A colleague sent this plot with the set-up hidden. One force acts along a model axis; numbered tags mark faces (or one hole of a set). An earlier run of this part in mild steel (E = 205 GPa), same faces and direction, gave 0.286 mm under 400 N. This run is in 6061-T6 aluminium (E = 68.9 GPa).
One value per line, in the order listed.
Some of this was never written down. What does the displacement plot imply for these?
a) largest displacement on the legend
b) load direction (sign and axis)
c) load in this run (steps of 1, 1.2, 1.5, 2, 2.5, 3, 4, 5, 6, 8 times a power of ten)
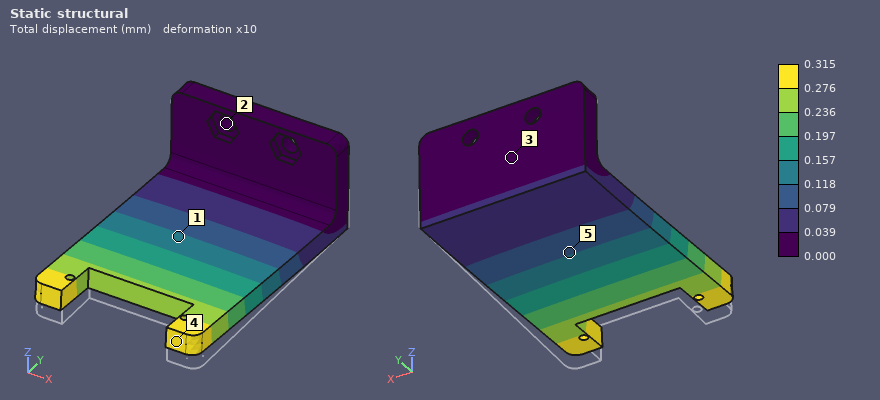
0.315 mm
+Z
150 N
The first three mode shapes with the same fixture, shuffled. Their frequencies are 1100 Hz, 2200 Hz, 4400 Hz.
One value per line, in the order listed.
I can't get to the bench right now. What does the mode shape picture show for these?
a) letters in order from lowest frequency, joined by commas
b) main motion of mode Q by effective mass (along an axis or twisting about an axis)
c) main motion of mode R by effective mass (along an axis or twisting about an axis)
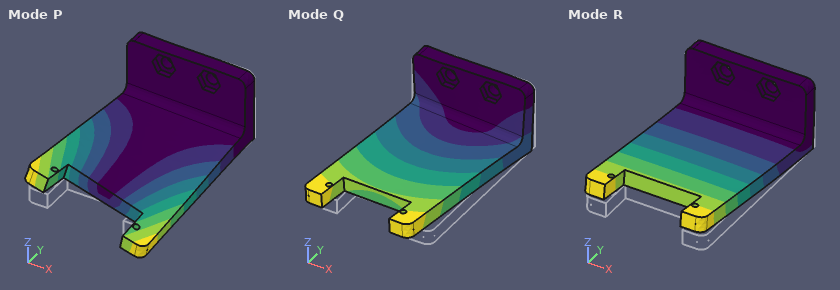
R, Q, P
along X
along Z
